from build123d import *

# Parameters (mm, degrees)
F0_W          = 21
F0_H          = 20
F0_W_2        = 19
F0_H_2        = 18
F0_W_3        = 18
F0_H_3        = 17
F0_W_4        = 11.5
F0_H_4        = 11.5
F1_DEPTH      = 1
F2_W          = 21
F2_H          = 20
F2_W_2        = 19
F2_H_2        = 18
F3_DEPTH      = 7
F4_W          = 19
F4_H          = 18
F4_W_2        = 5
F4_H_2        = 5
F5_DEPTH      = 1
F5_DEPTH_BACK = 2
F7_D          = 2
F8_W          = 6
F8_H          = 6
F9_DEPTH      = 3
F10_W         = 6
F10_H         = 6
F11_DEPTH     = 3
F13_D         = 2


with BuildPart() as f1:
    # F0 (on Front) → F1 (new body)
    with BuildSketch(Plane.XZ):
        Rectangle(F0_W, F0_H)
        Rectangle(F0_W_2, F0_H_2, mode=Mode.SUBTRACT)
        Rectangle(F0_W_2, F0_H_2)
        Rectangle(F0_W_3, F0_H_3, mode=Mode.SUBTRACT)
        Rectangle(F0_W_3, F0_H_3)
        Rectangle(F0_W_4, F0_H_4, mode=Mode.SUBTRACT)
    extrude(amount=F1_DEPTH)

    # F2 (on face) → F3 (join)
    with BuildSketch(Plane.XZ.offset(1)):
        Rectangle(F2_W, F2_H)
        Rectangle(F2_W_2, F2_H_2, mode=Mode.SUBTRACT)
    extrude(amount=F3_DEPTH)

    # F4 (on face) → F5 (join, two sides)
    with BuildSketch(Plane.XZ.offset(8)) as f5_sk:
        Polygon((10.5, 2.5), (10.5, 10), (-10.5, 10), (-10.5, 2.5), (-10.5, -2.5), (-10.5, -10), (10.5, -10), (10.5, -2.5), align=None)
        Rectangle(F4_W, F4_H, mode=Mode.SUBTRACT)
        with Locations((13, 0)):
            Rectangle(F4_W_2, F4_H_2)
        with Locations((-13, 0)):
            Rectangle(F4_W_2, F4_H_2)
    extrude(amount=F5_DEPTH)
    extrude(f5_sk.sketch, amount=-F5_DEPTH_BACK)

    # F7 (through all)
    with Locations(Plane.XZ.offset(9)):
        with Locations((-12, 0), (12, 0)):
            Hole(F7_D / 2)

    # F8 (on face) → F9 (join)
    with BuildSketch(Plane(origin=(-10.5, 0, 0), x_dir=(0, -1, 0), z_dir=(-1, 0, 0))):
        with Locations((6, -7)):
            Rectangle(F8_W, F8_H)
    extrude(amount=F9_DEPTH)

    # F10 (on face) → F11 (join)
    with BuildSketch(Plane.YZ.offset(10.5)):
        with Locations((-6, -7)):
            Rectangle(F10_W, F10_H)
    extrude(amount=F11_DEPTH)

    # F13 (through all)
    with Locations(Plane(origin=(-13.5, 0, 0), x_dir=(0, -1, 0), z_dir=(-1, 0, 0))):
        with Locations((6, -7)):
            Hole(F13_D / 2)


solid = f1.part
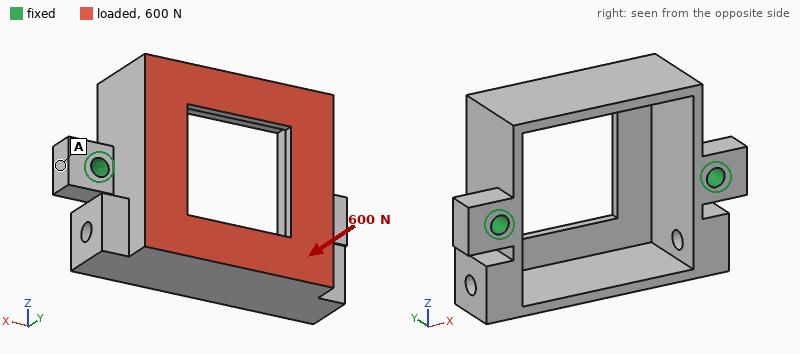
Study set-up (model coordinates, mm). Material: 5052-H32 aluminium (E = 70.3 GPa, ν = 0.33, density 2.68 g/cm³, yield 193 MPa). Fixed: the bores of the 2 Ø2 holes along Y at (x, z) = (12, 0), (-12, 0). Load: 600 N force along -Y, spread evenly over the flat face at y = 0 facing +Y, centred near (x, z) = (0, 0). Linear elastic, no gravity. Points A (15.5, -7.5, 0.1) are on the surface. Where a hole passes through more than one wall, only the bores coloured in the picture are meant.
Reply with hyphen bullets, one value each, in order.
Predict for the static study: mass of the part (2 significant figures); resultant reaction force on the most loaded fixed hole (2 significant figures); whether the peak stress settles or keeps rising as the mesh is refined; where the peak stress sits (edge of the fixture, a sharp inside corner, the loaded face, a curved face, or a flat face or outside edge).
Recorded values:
- 3.3 g
- 300 N
- keeps rising
- edge of the fixture
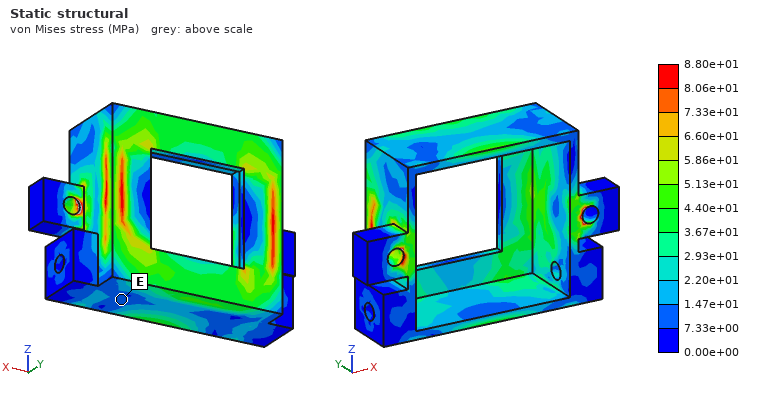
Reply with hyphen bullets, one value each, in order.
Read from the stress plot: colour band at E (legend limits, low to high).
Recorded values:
- 7.33e+00 to 1.47e+01 MPa
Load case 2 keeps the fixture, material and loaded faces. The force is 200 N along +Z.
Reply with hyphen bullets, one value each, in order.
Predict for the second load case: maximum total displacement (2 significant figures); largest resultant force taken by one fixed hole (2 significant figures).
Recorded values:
- 29 µm
- 100 N
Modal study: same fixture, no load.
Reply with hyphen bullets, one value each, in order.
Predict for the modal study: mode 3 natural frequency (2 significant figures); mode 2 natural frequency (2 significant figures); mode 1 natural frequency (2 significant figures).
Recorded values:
- 9700 Hz
- 9000 Hz
- 8800 Hz
